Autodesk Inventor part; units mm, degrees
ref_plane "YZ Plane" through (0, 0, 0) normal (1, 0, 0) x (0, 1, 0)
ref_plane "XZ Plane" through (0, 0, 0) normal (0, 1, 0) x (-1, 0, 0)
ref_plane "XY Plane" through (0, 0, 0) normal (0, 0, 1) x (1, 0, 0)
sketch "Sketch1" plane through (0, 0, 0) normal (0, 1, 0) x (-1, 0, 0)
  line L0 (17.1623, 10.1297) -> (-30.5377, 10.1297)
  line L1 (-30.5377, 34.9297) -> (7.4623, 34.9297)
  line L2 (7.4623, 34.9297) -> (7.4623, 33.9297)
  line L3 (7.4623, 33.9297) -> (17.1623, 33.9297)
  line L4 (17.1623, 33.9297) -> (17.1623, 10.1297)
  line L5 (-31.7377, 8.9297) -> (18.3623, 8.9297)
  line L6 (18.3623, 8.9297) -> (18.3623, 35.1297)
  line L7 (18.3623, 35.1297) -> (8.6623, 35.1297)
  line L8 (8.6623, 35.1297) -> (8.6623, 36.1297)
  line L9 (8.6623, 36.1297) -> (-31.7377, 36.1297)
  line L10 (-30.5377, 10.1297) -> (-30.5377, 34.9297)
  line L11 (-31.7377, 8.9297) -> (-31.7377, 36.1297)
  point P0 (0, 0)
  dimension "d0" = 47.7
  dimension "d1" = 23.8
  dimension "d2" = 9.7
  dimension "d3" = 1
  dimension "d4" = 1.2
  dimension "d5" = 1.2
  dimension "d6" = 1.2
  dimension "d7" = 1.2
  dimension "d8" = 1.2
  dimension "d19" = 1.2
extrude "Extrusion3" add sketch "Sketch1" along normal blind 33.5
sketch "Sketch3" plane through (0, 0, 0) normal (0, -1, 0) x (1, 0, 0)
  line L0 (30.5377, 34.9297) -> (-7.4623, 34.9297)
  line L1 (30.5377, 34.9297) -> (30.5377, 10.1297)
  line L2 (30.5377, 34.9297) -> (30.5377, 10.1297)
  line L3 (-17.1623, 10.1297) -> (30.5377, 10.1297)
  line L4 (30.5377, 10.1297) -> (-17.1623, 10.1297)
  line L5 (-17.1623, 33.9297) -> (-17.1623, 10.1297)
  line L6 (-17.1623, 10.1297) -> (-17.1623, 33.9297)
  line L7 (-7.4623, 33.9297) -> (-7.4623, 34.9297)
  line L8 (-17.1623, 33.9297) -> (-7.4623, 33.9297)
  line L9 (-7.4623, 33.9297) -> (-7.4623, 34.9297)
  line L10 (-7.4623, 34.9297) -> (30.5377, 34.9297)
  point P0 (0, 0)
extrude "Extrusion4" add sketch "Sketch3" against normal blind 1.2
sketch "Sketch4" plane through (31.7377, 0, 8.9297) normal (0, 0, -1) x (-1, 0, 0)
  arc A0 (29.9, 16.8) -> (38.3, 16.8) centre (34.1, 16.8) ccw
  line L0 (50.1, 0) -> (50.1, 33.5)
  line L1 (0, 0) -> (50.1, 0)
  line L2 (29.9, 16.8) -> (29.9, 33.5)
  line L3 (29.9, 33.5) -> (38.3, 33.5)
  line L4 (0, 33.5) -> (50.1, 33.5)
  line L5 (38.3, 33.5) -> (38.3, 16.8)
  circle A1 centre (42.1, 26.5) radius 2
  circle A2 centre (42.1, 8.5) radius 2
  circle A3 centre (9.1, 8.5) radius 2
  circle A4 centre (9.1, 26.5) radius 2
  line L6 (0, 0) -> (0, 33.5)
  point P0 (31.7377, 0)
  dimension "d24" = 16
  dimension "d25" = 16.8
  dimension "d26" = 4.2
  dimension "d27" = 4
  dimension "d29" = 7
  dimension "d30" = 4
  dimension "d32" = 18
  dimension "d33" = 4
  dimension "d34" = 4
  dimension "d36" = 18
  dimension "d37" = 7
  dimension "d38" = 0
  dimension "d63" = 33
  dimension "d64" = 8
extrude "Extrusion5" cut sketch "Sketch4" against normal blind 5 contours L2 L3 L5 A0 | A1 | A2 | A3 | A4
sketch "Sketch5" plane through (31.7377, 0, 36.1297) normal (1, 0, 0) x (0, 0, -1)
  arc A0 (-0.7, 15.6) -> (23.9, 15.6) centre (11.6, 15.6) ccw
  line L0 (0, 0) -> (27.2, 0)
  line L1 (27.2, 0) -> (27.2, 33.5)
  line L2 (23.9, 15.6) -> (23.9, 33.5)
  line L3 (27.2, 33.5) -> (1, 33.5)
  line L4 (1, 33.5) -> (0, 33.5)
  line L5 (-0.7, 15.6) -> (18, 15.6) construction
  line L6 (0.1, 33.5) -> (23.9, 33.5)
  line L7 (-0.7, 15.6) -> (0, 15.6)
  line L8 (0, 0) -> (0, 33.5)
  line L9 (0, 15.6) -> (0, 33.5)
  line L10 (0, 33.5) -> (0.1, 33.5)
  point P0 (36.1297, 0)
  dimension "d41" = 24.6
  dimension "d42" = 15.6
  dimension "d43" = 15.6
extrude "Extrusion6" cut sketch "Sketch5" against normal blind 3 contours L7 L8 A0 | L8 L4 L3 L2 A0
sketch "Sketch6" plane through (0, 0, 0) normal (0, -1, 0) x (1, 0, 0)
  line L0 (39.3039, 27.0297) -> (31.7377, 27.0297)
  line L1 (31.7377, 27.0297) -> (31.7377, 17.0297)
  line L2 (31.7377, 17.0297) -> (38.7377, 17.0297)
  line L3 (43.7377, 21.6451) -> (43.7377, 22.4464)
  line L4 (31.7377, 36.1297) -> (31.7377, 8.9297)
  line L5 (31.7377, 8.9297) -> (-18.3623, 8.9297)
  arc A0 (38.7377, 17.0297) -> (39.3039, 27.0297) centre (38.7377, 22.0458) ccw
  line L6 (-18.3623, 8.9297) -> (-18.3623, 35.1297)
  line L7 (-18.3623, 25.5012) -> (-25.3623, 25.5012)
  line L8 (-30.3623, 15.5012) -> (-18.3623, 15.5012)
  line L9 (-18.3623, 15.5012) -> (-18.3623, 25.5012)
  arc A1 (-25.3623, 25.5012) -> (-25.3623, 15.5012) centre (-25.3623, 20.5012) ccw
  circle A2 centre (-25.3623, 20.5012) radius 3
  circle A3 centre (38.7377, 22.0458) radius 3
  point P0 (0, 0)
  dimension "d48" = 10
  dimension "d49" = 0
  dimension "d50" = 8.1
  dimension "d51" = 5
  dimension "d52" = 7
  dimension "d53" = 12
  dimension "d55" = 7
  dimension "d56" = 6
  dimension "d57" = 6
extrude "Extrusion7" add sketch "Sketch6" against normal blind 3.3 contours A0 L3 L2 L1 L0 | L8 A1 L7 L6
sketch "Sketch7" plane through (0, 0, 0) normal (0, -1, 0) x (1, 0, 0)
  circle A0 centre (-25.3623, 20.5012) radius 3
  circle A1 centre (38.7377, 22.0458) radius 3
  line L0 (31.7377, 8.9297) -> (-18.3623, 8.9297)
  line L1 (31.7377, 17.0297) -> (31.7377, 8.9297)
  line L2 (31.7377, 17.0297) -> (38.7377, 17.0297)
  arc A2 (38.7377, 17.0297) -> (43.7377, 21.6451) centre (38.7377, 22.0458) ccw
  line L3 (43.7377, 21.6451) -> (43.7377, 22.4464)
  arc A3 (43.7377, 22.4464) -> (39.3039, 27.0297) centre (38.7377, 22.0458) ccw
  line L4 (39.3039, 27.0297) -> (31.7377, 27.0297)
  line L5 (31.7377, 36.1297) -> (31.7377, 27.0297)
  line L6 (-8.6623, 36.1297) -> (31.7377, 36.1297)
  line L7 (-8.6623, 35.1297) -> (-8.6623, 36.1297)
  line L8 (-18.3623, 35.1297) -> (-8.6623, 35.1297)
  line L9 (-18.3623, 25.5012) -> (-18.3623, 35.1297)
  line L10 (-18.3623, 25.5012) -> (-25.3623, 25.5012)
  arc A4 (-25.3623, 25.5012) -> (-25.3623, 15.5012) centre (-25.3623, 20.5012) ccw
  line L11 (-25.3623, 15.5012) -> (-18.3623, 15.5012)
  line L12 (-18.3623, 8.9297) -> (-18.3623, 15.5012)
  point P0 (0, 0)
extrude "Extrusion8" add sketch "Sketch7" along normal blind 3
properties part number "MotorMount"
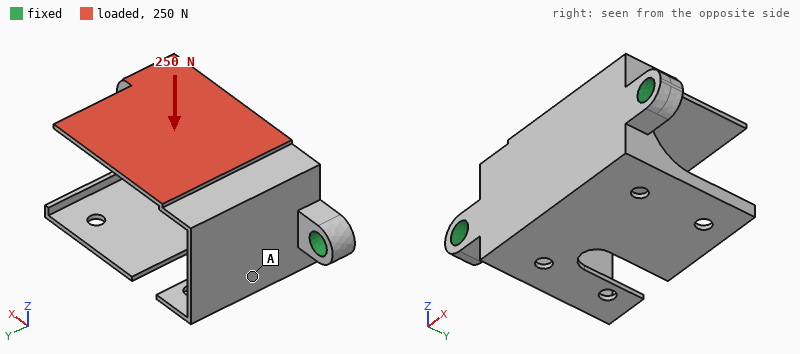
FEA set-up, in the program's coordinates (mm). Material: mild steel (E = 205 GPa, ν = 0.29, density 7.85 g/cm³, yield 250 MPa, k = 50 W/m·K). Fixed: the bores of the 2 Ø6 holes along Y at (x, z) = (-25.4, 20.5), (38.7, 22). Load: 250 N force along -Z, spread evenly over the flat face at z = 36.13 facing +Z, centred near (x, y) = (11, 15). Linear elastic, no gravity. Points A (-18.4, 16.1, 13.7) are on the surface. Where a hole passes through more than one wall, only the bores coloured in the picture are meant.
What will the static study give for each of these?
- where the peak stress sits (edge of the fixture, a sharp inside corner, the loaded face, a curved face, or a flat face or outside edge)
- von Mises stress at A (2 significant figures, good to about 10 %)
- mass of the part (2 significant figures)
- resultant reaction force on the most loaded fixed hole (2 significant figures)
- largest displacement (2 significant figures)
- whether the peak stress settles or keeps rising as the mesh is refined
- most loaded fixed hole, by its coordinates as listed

a sharp inside corner
20 MPa
90 g
150 N
0.41 mm
keeps rising
(38.7, 22)
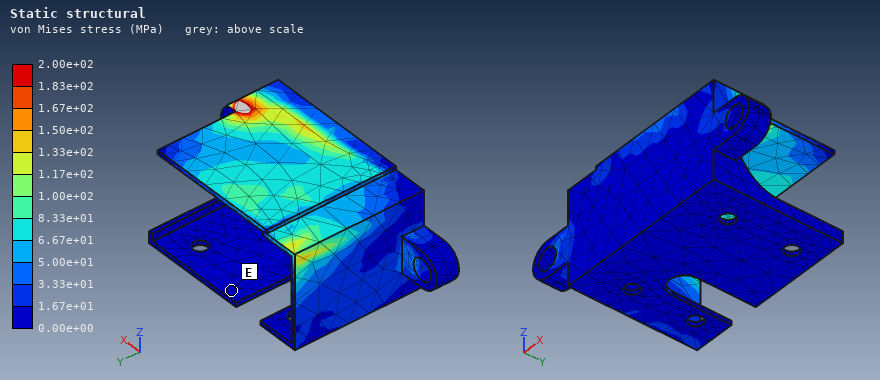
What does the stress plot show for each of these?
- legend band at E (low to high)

0.00e+00 to 1.67e+01 MPa
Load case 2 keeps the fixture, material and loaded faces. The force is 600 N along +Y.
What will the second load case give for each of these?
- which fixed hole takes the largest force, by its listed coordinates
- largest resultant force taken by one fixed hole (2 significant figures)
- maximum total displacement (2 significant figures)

(38.7, 22)
370 N
0.11 mm
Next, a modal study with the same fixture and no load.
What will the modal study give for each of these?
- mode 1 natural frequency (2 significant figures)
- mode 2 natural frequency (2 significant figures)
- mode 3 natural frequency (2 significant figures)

1500 Hz
1600 Hz
3400 Hz
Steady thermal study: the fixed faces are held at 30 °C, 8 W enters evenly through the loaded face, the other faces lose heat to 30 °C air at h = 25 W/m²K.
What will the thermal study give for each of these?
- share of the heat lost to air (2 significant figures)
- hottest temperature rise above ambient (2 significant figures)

38 %
45 K
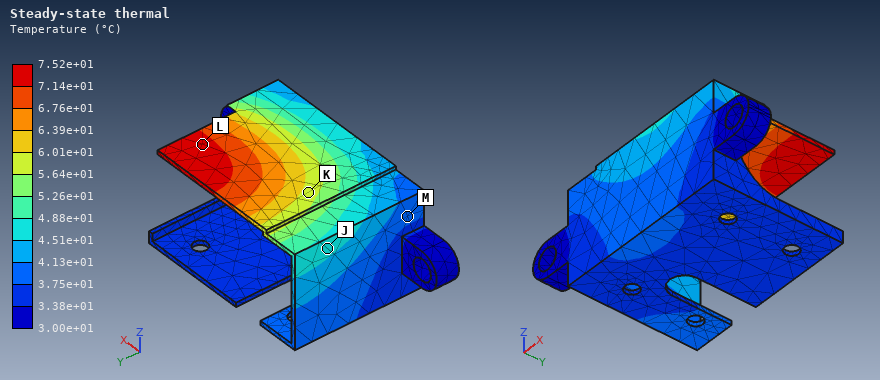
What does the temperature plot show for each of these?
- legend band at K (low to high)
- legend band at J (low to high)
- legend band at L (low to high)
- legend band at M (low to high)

5.64e+01 to 6.01e+01 °C
4.51e+01 to 4.88e+01 °C
7.14e+01 to 7.52e+01 °C
3.75e+01 to 4.13e+01 °C
